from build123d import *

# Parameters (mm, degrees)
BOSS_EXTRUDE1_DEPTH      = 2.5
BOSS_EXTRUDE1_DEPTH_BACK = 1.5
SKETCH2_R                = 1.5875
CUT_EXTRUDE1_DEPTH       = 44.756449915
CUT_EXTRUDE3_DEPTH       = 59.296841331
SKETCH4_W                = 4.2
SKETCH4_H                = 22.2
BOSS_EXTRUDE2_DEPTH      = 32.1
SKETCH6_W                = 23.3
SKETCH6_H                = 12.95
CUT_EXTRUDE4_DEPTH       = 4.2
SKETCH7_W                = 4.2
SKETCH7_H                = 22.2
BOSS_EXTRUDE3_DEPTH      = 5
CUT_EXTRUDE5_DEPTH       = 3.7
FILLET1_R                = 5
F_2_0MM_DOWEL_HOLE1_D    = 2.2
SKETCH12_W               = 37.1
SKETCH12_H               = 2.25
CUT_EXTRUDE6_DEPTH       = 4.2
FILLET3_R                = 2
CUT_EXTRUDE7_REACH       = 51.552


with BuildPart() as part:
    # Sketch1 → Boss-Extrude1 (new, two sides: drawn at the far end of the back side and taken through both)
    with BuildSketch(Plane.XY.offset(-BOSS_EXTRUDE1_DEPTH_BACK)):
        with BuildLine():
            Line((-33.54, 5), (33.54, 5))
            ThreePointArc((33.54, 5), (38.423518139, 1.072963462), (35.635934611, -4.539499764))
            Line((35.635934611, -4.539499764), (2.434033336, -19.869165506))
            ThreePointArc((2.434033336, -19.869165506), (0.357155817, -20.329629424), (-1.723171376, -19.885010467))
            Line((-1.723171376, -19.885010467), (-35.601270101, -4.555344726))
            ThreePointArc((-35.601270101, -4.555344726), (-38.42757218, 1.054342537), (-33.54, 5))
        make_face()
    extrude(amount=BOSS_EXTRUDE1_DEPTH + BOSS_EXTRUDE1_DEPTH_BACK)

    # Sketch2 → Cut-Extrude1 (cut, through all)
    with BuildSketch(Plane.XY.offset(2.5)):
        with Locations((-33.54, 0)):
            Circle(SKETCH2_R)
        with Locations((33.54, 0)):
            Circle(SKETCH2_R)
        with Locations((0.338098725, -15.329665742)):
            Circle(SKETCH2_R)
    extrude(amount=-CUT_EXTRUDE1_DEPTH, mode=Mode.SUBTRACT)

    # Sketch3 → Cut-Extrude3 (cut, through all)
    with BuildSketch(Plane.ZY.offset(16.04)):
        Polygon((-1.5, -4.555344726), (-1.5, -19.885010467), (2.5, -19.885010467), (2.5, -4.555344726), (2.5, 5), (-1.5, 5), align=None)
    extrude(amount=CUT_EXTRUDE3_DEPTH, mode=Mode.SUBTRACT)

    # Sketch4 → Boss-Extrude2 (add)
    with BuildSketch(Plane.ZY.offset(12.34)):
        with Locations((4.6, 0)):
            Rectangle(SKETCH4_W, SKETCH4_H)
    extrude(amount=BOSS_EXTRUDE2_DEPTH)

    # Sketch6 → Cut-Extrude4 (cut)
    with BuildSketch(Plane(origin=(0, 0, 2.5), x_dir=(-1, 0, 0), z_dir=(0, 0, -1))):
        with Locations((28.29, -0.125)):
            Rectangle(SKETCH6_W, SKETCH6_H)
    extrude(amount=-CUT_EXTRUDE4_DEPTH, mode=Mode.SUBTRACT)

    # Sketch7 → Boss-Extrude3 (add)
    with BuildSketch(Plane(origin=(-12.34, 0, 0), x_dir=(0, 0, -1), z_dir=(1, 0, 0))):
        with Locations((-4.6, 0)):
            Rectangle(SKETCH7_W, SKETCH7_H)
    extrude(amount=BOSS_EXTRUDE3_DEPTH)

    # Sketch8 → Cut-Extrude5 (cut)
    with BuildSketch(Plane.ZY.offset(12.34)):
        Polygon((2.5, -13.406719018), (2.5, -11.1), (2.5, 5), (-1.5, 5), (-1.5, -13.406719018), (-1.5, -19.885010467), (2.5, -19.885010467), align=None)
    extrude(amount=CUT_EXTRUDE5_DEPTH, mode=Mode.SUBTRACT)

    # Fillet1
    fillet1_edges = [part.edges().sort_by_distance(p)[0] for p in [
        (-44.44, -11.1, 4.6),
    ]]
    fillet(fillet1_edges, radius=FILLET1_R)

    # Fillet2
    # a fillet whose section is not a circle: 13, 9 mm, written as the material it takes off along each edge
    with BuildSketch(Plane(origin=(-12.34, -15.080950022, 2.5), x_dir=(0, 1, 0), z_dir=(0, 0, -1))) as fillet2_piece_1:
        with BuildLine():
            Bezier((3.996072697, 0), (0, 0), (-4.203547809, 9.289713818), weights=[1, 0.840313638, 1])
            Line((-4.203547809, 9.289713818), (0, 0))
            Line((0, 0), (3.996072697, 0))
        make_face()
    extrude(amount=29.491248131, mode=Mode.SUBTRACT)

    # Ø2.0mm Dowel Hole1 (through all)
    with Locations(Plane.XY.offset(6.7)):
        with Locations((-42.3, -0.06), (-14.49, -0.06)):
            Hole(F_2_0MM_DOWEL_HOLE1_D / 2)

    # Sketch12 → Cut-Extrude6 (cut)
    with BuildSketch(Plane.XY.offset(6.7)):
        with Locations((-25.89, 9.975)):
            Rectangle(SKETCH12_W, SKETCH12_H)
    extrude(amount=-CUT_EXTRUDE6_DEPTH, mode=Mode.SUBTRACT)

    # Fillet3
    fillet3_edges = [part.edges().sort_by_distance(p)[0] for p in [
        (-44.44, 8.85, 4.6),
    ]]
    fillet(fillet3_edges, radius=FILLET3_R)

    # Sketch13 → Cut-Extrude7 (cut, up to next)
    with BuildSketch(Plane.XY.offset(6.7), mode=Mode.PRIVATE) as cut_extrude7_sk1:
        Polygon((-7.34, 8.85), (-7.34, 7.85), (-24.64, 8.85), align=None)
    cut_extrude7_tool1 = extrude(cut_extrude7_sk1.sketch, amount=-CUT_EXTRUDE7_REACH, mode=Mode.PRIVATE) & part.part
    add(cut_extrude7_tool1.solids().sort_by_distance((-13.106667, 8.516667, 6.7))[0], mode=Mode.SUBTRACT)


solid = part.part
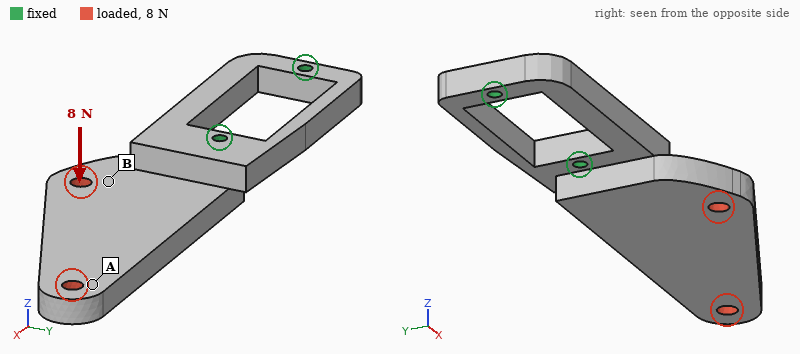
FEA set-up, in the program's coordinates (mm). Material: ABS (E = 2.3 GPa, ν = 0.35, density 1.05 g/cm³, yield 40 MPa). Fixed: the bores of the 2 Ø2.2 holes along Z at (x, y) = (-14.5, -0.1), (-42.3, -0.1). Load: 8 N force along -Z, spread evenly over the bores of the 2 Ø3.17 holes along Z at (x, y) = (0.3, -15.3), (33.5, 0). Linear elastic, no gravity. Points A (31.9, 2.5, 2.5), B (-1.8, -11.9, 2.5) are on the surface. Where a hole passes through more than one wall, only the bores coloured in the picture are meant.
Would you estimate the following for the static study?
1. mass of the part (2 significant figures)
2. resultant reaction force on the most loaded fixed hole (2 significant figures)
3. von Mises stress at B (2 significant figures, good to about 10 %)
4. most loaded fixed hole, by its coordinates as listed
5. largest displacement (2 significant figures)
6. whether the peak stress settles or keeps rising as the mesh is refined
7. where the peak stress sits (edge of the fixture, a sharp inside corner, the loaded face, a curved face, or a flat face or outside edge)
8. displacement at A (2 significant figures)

5.7 g
10 N
2.0 MPa
(-14.5, -0.1)
0.88 mm
keeps rising
edge of the fixture
0.72 mm
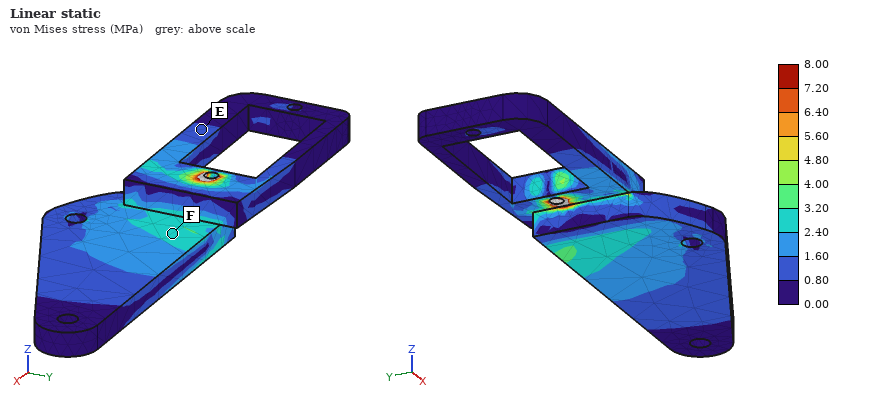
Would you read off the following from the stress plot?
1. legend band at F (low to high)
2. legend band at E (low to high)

2.40 to 3.20 MPa
0.80 to 1.60 MPa
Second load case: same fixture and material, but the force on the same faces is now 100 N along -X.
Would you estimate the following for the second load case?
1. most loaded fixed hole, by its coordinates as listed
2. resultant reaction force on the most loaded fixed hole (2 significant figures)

(-14.5, -0.1)
84 N
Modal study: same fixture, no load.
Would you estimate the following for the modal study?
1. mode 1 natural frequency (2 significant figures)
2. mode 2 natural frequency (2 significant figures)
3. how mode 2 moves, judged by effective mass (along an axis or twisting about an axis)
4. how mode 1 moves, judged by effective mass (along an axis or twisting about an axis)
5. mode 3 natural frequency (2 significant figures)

410 Hz
790 Hz
along Y
along Z
1500 Hz
